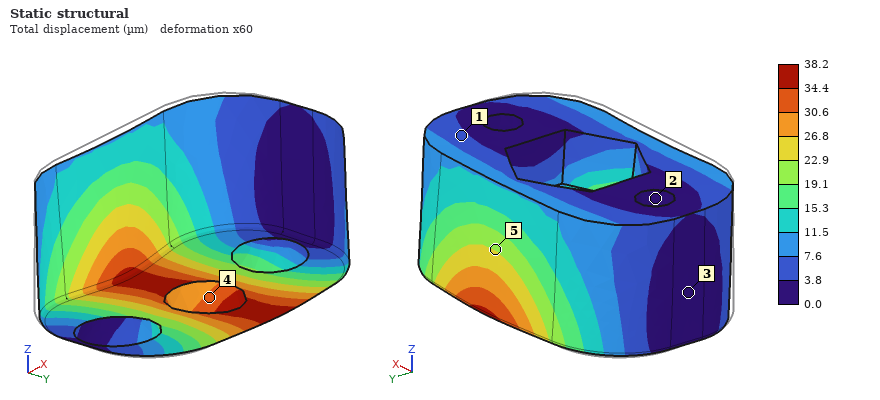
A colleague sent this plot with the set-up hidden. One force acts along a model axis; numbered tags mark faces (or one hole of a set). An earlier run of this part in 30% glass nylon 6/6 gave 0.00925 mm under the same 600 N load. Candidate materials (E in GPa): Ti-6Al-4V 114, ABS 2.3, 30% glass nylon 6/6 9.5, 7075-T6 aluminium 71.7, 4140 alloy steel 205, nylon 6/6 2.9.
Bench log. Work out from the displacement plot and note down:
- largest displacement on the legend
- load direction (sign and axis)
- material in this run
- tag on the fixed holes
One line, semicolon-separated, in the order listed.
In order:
38.2 µm; +Y; ABS; 2
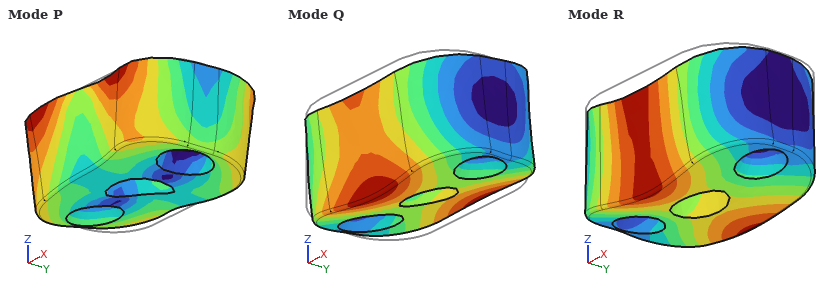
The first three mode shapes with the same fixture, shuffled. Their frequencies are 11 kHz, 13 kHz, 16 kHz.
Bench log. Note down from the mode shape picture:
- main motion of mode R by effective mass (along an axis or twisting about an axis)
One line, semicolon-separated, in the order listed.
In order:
along Z
